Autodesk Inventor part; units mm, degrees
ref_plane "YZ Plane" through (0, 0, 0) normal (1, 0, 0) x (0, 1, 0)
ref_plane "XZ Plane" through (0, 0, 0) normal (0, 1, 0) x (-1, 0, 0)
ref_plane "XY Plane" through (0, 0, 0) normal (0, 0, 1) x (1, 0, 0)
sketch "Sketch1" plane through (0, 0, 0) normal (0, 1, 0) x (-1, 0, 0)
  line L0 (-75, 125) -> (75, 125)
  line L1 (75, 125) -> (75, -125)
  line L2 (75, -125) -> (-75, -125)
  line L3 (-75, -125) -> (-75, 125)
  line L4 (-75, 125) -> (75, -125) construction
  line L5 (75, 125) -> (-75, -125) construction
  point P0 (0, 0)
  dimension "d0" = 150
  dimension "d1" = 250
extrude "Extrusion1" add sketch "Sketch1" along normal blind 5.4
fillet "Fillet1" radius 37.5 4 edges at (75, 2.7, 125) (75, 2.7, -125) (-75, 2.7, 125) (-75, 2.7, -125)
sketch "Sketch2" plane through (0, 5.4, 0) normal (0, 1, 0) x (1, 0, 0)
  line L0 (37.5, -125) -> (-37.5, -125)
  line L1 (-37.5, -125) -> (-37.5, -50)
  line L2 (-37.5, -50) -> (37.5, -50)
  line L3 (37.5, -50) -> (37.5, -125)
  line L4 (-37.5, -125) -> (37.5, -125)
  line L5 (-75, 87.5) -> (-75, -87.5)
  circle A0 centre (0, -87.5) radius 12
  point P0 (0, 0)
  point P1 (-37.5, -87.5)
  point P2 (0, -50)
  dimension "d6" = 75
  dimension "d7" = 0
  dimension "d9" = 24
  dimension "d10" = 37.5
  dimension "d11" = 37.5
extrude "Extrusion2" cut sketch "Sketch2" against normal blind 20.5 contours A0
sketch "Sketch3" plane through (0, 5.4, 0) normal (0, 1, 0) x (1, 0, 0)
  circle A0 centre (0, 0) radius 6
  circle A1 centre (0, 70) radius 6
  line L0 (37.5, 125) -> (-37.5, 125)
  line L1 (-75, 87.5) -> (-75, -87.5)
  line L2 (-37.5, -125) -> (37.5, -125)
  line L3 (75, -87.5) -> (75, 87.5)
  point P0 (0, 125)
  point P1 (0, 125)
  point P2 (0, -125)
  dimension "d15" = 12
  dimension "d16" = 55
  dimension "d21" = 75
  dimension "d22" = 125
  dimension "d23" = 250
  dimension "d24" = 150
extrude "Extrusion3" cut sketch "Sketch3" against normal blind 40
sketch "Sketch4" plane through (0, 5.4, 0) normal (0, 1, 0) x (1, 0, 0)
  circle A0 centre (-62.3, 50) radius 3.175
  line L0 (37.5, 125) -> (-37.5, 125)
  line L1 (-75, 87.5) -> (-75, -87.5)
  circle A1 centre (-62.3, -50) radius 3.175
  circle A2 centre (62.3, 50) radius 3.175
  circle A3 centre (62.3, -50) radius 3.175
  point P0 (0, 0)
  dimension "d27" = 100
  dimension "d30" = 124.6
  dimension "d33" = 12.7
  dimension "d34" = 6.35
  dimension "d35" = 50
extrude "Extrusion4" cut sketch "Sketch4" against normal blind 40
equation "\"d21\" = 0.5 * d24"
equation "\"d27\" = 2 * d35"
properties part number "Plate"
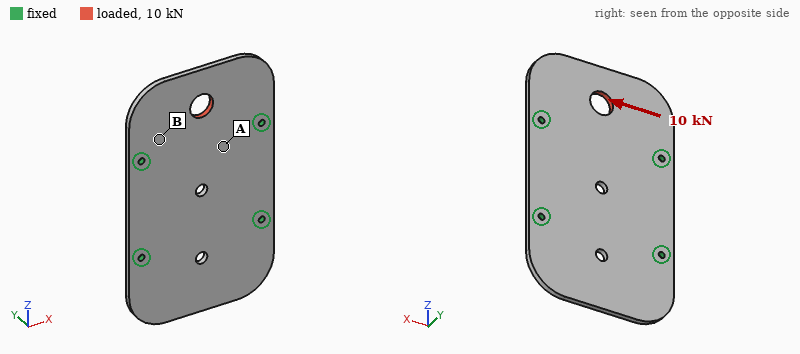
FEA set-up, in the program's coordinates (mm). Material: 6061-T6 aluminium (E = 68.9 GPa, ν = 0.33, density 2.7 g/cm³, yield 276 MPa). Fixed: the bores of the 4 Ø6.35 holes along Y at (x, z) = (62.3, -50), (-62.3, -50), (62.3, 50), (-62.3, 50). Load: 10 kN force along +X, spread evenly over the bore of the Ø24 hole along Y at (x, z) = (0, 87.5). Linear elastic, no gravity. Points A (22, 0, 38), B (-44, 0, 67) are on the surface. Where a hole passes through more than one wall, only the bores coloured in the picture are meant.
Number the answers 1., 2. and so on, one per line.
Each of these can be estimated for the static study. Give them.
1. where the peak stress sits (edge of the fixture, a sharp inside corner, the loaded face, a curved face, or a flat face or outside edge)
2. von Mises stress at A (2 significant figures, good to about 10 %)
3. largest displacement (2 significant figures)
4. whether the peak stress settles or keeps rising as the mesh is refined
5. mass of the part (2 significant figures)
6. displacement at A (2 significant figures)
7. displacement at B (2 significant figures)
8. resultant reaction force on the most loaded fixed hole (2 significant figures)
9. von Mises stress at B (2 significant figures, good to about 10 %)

1. edge of the fixture
2. 8.5 MPa
3. 44 µm
4. keeps rising
5. 520 g
6. 8.4 µm
7. 16 µm
8. 5.4 kN
9. 27 MPa
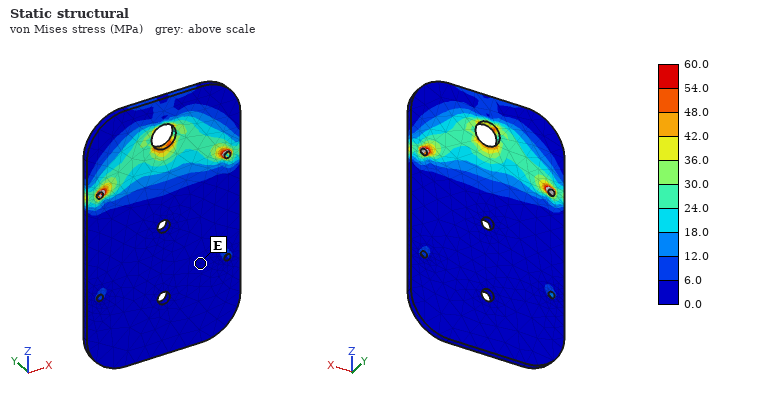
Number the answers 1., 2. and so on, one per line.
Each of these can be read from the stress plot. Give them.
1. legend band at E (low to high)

1. 0.0 to 6.0 MPa
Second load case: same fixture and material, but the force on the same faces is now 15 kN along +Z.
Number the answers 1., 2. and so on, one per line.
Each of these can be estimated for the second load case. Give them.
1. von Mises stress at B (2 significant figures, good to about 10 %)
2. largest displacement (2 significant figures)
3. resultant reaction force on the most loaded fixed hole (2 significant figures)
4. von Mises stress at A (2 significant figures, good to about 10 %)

1. 26 MPa
2. 51 µm
3. 5.3 kN
4. 19 MPa
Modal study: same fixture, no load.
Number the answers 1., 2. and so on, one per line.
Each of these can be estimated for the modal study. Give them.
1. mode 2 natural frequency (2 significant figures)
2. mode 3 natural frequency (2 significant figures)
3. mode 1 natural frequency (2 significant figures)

1. 670 Hz
2. 1400 Hz
3. 660 Hz
